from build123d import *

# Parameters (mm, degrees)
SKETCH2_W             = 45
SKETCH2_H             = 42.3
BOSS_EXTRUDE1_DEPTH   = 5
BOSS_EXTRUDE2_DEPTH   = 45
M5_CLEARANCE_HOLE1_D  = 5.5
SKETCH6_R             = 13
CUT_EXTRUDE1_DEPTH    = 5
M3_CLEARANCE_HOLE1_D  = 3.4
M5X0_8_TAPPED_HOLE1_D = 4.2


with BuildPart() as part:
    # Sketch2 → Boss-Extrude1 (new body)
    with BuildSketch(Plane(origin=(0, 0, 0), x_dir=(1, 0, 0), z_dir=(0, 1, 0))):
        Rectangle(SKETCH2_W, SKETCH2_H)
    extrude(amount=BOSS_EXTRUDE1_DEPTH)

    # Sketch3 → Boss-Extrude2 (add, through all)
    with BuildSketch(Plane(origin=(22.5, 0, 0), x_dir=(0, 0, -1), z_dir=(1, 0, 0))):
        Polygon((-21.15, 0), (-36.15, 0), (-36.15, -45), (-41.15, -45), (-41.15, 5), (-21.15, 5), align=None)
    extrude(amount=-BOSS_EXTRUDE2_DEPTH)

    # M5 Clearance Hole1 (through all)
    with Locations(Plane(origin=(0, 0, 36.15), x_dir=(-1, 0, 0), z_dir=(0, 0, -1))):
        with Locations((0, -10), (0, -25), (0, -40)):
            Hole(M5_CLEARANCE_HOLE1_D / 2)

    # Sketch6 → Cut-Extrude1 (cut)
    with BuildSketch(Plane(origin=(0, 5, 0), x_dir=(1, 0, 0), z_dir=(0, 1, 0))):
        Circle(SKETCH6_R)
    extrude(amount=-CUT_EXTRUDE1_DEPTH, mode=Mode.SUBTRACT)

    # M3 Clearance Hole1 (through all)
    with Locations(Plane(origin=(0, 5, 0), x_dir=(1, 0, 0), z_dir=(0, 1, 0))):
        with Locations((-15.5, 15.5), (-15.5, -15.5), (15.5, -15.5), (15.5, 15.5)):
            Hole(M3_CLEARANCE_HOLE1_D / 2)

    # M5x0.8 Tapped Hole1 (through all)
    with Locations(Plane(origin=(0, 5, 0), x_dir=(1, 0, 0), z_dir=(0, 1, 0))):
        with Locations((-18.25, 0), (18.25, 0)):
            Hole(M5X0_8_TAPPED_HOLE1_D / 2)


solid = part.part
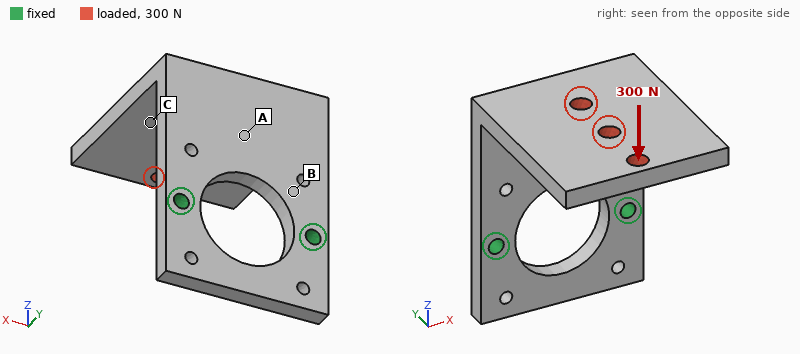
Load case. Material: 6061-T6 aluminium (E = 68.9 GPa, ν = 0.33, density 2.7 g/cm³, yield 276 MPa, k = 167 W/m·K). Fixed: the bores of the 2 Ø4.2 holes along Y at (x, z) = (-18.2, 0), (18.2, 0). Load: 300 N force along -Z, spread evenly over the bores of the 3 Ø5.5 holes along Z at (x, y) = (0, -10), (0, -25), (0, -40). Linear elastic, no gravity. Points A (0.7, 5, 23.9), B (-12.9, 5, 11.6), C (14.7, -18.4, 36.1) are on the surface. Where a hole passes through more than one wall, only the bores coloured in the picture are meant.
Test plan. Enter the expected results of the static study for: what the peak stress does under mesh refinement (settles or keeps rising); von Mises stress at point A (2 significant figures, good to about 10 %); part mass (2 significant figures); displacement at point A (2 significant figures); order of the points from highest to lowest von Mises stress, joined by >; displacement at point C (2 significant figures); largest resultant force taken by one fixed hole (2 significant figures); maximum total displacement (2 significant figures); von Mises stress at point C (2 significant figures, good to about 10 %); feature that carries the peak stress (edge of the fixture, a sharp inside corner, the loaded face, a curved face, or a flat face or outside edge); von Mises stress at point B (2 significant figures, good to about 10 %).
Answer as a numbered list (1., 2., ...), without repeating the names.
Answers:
1. keeps rising
2. 33 MPa
3. 56 g
4. 0.14 mm
5. B > A > C
6. 0.41 mm
7. 160 N
8. 0.85 mm
9. 16 MPa
10. edge of the fixture
11. 76 MPa
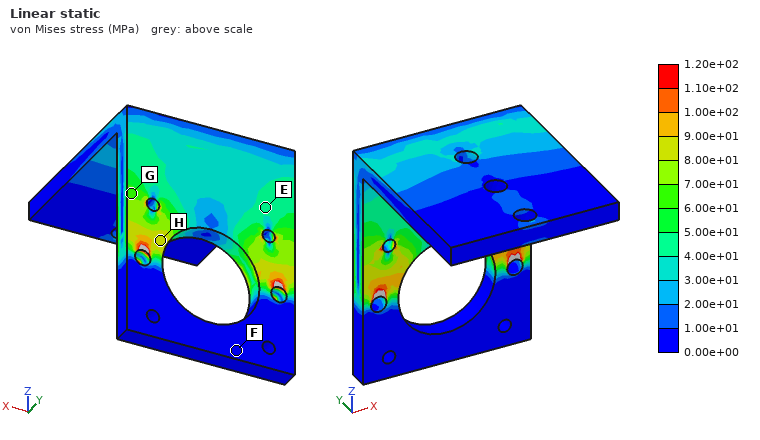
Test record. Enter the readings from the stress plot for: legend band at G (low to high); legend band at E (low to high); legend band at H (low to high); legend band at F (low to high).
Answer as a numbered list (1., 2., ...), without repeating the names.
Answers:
1. 6.00e+01 to 7.00e+01 MPa
2. 4.00e+01 to 5.00e+01 MPa
3. 8.00e+01 to 9.00e+01 MPa
4. 0.00e+00 to 1.00e+01 MPa
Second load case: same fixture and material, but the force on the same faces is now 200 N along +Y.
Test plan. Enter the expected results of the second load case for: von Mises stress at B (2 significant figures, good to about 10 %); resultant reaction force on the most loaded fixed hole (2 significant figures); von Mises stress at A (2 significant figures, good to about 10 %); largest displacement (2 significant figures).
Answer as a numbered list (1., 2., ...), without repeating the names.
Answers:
1. 50 MPa
2. 100 N
3. 12 MPa
4. 0.42 mm
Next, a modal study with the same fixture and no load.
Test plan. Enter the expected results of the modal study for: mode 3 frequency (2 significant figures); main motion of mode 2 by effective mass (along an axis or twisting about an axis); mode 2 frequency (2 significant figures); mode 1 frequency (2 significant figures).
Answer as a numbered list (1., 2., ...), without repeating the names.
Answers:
1. 1900 Hz
2. along X
3. 1300 Hz
4. 610 Hz
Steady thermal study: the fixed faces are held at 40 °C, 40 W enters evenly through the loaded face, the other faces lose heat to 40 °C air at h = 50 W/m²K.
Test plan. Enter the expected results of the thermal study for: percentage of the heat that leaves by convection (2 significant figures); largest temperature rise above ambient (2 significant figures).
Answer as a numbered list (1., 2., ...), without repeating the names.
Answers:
1. 40 %
2. 62 K
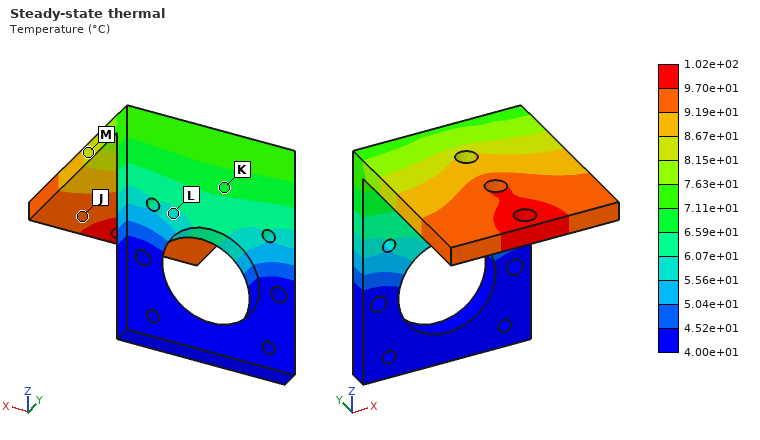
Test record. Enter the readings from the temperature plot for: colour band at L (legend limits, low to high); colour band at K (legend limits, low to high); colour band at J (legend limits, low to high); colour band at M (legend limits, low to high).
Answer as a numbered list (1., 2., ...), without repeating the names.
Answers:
1. 5.56e+01 to 6.07e+01 °C
2. 6.59e+01 to 7.11e+01 °C
3. 9.19e+01 to 9.70e+01 °C
4. 8.15e+01 to 8.67e+01 °C
